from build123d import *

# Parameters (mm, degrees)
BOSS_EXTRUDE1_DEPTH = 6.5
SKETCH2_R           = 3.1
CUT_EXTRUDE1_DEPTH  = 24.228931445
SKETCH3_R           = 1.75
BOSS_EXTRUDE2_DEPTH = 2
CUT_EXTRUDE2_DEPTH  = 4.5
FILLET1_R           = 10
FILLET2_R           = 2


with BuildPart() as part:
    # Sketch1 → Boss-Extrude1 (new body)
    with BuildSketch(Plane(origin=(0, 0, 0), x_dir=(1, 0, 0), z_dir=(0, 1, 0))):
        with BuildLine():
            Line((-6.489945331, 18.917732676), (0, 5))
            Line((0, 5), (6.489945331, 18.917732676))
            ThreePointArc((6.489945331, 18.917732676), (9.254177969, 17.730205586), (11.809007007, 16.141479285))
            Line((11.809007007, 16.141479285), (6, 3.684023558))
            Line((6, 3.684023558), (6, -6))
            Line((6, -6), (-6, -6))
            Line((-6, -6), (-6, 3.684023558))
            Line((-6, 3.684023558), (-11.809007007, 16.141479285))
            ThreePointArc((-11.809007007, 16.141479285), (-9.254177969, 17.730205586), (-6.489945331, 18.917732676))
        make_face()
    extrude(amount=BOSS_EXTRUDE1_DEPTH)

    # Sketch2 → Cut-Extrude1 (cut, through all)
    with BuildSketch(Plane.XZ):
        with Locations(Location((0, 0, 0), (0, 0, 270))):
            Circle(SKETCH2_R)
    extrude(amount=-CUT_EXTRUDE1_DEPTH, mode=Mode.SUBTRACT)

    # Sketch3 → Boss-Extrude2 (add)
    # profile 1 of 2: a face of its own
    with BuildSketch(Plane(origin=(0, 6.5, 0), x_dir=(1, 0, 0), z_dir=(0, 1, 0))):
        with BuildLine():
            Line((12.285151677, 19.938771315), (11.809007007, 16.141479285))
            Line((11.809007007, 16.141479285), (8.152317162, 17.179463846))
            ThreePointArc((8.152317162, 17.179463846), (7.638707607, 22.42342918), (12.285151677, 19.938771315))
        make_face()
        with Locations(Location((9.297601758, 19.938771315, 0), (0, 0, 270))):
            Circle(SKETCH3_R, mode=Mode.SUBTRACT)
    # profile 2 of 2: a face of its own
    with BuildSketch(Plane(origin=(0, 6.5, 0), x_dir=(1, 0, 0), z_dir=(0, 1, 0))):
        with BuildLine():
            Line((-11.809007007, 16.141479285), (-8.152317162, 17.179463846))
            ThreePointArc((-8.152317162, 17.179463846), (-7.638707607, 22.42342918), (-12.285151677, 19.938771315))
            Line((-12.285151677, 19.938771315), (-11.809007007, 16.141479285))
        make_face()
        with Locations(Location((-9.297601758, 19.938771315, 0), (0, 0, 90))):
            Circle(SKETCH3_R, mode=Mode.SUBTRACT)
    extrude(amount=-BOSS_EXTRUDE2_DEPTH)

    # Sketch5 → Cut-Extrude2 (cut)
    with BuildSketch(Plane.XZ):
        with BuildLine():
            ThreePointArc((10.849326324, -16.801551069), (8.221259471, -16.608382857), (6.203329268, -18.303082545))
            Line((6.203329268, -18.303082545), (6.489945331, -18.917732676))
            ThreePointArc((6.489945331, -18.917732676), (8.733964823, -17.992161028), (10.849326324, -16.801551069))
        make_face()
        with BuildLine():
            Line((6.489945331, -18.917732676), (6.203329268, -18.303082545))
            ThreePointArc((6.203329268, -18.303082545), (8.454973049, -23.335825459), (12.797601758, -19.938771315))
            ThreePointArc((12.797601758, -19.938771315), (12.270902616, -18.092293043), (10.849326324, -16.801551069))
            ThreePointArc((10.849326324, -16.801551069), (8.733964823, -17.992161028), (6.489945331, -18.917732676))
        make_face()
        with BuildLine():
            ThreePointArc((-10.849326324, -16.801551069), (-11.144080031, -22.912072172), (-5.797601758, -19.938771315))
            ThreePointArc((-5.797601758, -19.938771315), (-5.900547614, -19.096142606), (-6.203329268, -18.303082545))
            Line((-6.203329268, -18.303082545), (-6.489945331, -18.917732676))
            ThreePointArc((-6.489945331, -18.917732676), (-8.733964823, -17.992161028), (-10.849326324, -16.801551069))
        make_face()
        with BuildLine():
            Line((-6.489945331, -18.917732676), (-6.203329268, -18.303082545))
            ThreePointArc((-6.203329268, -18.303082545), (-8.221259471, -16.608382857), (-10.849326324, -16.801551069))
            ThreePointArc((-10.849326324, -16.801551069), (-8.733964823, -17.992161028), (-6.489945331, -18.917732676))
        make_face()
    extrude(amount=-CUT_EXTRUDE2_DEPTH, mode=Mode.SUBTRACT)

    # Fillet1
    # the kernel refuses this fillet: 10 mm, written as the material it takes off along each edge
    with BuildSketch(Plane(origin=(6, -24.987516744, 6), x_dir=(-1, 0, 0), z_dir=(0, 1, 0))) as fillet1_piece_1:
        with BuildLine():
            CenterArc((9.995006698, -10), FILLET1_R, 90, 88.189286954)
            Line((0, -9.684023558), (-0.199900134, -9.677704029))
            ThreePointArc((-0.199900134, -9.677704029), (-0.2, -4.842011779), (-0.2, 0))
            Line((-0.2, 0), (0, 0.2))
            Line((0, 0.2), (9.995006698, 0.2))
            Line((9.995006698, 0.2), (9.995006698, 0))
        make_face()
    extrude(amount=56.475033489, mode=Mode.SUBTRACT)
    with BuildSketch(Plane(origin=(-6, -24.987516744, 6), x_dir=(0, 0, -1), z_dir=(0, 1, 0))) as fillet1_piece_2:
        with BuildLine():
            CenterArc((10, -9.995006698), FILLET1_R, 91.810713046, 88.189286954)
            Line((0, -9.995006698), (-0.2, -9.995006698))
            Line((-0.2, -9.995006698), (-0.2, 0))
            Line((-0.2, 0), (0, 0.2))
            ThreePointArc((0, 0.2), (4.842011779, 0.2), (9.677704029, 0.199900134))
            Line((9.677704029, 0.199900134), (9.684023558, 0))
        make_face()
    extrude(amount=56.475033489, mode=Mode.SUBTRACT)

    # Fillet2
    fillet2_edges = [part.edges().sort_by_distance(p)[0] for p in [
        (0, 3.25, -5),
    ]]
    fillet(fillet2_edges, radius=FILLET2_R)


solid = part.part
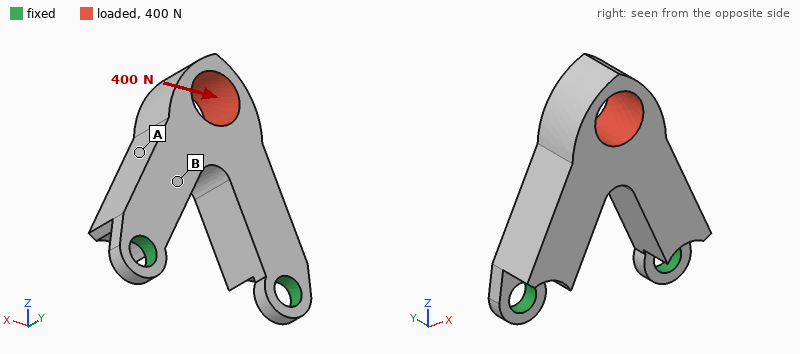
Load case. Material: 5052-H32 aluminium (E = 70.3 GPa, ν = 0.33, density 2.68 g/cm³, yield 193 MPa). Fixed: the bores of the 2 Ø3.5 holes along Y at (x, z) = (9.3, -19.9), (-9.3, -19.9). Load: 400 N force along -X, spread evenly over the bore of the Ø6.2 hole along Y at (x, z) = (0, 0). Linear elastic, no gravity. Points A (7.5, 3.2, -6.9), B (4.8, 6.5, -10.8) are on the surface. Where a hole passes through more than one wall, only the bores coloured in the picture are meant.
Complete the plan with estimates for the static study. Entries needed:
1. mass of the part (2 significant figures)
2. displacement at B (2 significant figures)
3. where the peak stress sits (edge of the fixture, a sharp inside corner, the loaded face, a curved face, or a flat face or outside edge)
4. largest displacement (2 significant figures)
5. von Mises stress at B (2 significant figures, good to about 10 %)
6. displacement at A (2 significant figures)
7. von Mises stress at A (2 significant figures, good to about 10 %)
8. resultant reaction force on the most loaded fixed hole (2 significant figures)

4.1 g
6.7 µm
edge of the fixture
21 µm
23 MPa
9.1 µm
9.1 MPa
420 N
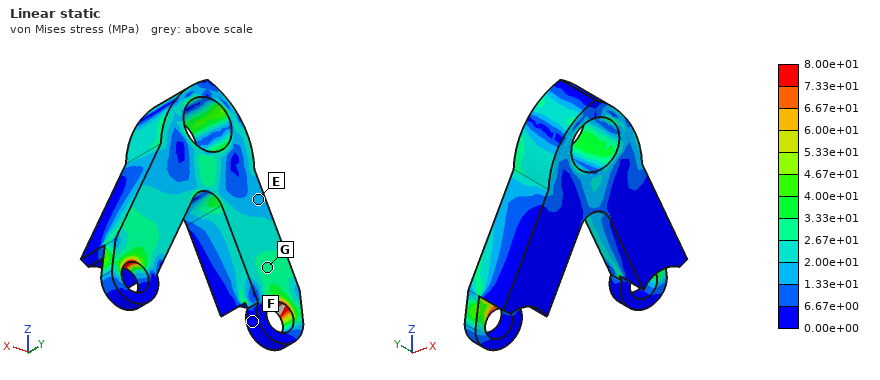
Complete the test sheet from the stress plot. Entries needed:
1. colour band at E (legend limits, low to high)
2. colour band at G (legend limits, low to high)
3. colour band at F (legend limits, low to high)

1.33e+01 to 2.00e+01 MPa
2.67e+01 to 3.33e+01 MPa
0.00e+00 to 6.67e+00 MPa
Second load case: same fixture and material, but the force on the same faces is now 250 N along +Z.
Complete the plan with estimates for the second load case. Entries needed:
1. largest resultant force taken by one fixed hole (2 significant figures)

130 N
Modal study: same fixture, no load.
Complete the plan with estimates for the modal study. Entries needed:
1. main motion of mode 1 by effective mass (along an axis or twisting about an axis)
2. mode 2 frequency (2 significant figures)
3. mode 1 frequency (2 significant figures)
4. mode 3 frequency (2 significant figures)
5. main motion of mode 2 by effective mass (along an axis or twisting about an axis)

along Y
20 kHz
3300 Hz
21 kHz
along X
